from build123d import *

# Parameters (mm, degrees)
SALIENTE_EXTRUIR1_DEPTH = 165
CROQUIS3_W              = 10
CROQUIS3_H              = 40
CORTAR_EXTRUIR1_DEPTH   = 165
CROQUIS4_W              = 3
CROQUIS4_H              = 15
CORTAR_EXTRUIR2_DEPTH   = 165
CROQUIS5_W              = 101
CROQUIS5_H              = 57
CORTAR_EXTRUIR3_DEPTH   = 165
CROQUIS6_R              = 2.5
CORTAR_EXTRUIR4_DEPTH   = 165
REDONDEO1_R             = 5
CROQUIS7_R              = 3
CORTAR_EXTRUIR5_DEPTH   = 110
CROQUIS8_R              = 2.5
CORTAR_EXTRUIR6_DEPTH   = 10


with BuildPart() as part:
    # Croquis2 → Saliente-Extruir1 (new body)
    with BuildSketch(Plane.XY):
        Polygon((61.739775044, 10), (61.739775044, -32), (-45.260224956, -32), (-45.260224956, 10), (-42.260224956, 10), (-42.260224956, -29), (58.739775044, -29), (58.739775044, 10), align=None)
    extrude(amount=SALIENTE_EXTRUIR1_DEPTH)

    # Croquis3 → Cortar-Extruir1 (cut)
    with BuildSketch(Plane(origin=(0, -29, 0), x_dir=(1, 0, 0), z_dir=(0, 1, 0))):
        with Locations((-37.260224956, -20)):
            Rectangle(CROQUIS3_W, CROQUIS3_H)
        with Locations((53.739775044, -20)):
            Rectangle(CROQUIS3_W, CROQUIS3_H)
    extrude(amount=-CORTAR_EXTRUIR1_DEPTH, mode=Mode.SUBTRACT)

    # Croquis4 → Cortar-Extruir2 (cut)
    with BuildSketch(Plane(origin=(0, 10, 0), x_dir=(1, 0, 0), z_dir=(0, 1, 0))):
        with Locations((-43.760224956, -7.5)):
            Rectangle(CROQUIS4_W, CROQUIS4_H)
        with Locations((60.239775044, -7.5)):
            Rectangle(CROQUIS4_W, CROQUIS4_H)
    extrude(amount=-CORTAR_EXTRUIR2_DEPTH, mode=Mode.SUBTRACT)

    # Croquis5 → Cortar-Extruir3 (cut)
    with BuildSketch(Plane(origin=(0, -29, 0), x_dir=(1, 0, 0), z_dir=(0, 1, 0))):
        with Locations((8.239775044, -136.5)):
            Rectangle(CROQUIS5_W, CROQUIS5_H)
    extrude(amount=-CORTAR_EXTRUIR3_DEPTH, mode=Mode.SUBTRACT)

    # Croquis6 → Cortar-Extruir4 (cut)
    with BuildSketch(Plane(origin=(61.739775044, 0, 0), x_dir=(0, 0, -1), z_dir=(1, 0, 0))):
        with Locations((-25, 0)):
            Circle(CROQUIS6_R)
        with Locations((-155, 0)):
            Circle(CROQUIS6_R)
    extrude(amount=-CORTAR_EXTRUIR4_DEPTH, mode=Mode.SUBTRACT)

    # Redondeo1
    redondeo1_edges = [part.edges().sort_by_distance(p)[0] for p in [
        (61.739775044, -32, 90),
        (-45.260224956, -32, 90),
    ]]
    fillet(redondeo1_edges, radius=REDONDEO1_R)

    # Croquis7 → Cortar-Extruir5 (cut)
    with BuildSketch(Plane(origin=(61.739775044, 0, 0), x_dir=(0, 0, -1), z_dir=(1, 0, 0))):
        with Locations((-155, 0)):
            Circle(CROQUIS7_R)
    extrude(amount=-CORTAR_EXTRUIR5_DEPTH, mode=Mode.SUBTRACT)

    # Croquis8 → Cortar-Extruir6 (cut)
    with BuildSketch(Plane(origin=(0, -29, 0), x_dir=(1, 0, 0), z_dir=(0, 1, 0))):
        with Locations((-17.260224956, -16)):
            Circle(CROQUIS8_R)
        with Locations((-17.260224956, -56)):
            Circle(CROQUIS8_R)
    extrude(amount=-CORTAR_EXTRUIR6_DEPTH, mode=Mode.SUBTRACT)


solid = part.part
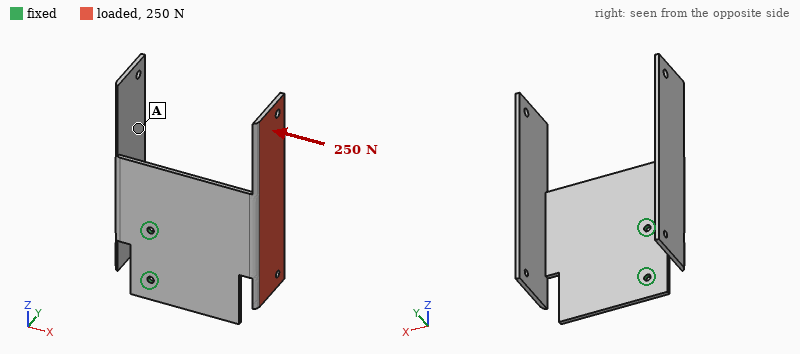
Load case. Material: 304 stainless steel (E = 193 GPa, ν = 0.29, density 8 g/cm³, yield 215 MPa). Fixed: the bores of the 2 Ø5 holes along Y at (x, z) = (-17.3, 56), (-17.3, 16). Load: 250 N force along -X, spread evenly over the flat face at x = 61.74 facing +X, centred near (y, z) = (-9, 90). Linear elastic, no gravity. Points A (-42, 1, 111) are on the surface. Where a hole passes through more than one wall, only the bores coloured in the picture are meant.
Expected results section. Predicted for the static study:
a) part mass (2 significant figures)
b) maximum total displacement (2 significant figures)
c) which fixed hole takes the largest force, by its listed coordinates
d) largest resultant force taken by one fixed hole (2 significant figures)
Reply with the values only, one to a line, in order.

530 g
1.1 mm
(-17.3, 56)
440 N
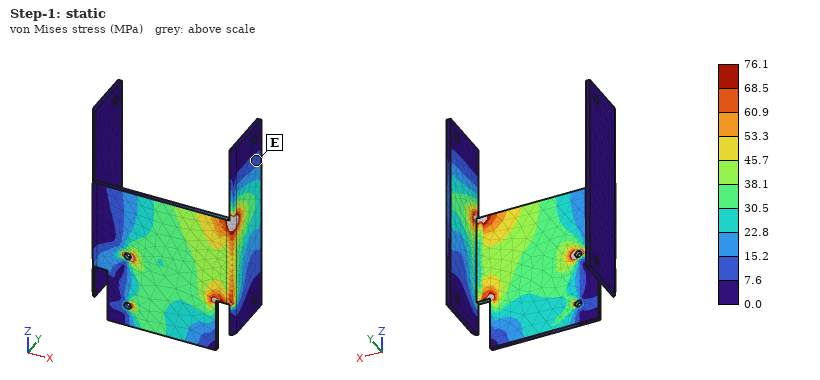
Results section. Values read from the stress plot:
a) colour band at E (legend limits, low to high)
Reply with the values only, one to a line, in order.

7.6 to 15.2 MPa
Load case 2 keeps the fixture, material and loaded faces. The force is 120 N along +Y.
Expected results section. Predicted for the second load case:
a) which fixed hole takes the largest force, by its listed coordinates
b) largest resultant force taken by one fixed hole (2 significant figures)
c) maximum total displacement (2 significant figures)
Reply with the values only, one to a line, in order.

(-17.3, 56)
170 N
1.2 mm
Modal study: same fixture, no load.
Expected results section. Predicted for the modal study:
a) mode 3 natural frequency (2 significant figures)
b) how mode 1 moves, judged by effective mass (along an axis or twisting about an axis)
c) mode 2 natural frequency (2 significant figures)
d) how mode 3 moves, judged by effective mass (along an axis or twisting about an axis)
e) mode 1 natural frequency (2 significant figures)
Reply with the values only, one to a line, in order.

300 Hz
along Y
260 Hz
along Y
140 Hz
